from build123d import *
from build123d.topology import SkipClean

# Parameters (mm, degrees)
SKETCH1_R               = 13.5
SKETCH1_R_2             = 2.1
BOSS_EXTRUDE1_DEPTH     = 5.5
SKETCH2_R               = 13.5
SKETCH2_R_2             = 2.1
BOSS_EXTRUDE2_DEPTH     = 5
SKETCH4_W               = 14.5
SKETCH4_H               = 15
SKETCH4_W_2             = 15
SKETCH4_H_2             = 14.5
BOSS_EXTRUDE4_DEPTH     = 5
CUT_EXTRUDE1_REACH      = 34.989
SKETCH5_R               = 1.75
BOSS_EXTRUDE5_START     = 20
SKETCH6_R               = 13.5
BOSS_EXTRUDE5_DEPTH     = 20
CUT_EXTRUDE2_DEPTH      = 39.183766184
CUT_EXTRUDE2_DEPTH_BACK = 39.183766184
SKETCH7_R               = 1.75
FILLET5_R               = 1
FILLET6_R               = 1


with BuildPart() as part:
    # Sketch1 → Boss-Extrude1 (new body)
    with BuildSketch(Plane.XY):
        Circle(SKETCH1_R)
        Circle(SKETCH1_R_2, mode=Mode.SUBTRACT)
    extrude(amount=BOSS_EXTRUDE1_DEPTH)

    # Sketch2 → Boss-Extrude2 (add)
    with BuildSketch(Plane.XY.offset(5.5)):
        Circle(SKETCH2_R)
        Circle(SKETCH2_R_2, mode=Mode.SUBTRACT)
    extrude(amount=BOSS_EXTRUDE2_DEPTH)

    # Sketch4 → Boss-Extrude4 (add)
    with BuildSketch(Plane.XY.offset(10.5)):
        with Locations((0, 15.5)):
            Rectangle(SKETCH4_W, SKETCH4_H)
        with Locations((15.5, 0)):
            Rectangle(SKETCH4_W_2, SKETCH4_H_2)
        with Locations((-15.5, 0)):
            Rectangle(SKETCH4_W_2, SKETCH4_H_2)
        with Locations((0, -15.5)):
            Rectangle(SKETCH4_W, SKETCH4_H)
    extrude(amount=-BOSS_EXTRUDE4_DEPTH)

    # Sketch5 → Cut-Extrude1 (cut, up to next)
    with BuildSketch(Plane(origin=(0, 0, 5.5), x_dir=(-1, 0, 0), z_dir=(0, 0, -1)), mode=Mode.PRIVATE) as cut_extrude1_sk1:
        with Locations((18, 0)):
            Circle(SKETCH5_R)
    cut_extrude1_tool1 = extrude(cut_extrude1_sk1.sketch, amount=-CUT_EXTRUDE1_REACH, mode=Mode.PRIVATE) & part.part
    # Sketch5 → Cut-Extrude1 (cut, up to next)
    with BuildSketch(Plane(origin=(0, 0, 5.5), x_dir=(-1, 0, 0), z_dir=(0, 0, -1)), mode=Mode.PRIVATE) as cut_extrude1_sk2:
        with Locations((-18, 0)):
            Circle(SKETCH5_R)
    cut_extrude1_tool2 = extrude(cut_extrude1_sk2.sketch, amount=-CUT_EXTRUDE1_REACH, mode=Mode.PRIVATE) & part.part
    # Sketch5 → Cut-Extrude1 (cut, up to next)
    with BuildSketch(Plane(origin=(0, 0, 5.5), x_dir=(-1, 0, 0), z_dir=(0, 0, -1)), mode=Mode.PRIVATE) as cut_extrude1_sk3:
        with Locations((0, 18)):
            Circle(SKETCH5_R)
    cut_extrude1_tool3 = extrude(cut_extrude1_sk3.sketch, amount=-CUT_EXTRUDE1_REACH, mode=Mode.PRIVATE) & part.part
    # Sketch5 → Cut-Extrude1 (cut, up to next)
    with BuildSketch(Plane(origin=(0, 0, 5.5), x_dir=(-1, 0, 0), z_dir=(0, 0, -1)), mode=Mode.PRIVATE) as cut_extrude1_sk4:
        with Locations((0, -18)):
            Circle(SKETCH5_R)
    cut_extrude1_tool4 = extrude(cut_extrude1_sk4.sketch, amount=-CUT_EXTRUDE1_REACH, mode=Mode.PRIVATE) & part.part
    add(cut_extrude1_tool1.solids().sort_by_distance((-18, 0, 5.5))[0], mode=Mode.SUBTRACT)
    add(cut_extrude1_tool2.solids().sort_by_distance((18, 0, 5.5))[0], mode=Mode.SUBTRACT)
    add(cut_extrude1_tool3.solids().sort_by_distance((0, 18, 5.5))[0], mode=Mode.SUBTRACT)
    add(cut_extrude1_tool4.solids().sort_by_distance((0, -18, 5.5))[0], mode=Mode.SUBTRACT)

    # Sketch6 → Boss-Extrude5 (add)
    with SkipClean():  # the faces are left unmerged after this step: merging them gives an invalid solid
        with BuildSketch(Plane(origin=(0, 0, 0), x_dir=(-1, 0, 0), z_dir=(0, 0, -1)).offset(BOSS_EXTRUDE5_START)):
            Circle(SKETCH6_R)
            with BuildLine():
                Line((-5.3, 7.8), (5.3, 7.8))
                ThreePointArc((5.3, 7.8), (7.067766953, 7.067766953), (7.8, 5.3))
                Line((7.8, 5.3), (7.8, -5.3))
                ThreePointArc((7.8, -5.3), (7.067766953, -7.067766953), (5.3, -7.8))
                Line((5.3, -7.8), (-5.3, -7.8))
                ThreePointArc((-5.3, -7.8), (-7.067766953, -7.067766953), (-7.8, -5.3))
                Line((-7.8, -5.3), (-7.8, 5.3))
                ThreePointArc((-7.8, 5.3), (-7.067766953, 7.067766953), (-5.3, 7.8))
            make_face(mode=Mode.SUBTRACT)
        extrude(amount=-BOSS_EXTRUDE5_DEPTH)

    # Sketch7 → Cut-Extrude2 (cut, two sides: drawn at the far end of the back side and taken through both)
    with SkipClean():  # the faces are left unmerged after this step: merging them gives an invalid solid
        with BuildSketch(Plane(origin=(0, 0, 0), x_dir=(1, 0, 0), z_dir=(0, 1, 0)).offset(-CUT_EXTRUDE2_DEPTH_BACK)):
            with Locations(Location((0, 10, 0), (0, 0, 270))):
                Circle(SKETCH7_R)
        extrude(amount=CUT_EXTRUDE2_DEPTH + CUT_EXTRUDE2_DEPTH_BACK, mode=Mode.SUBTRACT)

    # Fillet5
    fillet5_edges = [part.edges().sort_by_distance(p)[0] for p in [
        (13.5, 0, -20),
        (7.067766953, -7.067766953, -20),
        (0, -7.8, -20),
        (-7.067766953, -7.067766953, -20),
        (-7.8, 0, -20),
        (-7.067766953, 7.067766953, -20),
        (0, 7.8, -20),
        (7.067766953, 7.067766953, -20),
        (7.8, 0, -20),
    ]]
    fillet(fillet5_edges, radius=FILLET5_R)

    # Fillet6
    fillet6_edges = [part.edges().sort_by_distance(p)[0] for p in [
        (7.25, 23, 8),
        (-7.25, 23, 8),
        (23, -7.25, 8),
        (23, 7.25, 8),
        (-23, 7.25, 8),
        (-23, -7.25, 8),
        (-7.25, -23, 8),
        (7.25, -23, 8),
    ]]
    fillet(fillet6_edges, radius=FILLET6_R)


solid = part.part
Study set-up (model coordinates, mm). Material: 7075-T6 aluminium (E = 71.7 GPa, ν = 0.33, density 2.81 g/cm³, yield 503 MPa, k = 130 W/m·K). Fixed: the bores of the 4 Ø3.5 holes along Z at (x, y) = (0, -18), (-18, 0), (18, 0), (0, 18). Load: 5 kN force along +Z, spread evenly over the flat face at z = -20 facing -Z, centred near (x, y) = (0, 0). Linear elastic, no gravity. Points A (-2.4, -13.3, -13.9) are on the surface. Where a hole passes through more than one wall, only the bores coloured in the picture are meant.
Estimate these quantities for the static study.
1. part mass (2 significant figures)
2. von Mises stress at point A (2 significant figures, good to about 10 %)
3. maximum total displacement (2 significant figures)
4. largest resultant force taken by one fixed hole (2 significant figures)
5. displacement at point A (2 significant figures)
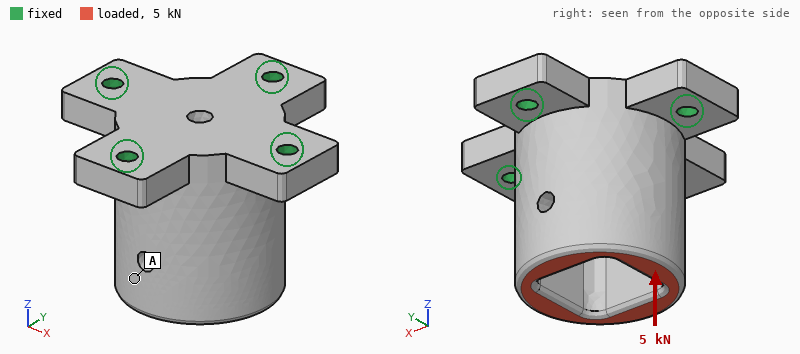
43 g
18 MPa
15 µm
1.3 kN
13 µm
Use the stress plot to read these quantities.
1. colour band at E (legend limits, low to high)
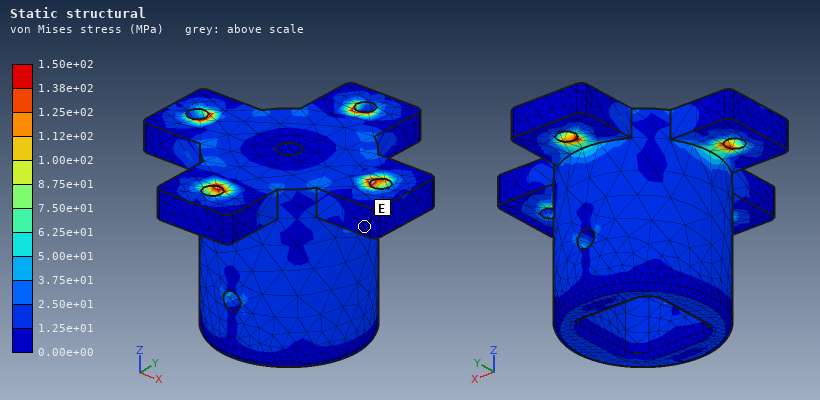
0.00e+00 to 1.25e+01 MPa
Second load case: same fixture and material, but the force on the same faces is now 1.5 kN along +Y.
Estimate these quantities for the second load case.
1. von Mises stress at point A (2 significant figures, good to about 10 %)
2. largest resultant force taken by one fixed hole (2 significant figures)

15 MPa
1.4 kN
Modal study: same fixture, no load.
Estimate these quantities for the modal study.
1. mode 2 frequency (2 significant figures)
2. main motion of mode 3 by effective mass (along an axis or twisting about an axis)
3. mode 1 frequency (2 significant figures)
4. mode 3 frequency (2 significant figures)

12 kHz
along Z
12 kHz
19 kHz
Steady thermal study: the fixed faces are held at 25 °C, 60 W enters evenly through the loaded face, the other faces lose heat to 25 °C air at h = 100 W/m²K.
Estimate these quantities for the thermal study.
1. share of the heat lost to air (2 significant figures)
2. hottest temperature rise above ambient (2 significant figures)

18 %
44 K
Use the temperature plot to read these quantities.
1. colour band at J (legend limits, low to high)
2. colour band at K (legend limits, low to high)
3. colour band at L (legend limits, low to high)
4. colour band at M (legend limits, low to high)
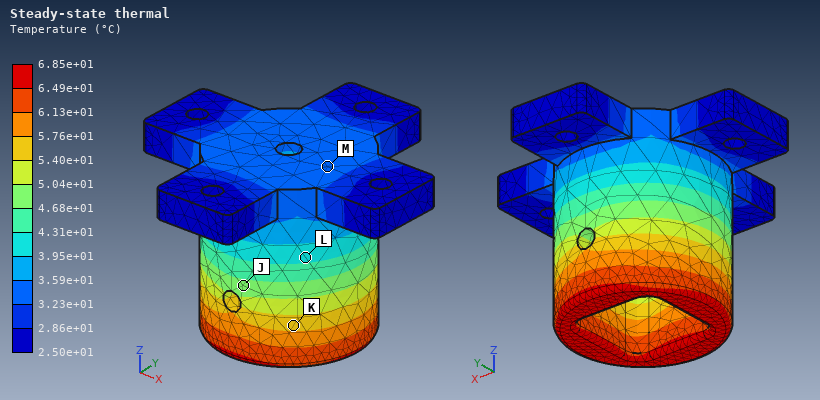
4.68e+01 to 5.04e+01 °C
5.40e+01 to 5.76e+01 °C
3.95e+01 to 4.31e+01 °C
3.23e+01 to 3.59e+01 °C
